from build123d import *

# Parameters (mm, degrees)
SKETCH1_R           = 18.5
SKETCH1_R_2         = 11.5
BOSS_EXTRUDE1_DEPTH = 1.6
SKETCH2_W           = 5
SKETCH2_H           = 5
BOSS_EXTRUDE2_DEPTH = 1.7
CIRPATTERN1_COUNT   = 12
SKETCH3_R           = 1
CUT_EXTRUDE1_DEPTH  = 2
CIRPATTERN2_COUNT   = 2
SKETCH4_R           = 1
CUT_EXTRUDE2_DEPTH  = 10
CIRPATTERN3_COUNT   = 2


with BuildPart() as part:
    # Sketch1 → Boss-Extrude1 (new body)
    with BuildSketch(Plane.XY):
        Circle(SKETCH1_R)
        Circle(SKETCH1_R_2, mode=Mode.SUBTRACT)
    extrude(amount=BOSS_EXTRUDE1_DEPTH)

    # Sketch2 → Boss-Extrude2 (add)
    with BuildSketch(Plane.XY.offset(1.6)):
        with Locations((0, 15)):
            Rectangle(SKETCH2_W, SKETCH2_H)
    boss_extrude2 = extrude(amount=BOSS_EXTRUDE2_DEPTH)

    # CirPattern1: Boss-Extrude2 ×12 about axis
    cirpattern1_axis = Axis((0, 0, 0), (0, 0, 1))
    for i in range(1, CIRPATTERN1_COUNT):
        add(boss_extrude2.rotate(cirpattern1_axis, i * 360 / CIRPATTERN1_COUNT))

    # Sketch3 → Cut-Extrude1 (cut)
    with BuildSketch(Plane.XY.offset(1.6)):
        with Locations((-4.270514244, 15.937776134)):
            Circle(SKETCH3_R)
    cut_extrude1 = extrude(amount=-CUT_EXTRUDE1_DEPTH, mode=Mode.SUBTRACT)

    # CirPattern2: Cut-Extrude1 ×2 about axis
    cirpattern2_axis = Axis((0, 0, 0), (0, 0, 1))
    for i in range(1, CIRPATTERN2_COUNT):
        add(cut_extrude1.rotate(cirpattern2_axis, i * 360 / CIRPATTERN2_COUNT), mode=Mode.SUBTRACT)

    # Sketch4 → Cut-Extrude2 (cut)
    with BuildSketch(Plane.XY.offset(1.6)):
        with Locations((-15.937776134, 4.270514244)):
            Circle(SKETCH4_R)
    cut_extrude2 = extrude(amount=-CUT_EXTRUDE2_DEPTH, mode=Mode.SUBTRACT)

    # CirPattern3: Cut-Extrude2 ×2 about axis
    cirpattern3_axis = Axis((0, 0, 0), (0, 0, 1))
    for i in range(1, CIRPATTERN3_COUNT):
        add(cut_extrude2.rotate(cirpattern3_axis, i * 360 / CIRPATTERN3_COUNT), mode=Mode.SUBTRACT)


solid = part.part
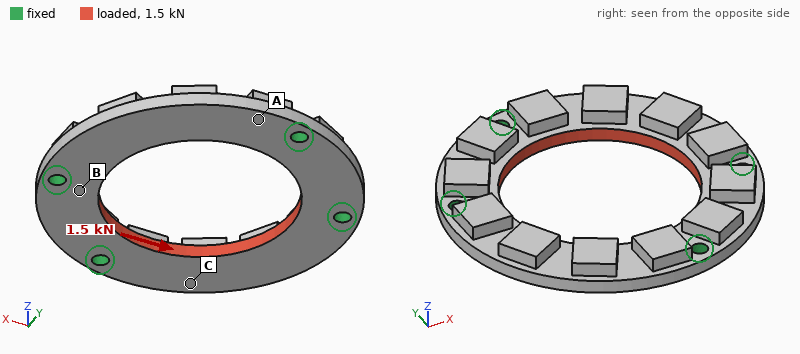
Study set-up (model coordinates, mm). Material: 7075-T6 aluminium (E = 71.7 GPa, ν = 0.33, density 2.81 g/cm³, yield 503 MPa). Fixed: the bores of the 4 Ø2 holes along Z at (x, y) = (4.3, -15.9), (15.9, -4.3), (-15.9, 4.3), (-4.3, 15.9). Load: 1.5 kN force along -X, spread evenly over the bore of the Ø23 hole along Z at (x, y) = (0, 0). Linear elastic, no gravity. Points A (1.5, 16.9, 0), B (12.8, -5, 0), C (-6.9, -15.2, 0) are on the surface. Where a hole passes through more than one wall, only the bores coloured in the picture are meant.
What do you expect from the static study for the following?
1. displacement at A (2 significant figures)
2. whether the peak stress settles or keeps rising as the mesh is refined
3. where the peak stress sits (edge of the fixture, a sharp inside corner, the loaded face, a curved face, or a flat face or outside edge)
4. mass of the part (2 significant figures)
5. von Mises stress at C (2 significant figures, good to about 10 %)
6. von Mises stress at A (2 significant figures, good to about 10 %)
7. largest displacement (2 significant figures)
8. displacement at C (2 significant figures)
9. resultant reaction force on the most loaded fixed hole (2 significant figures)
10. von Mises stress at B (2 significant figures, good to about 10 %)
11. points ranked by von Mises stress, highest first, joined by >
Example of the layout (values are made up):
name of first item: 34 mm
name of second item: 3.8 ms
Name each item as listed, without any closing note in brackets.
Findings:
displacement at A: 2.1 µm
whether the peak stress settles or keeps rising as the mesh is refined: keeps rising
where the peak stress sits: edge of the fixture
mass of the part: 4.3 g
von Mises stress at C: 18 MPa
von Mises stress at A: 26 MPa
largest displacement: 8.5 µm
displacement at C: 4.5 µm
resultant reaction force on the most loaded fixed hole: 430 N
von Mises stress at B: 39 MPa
points ranked by von Mises stress, highest first, joined by >: B > A > C
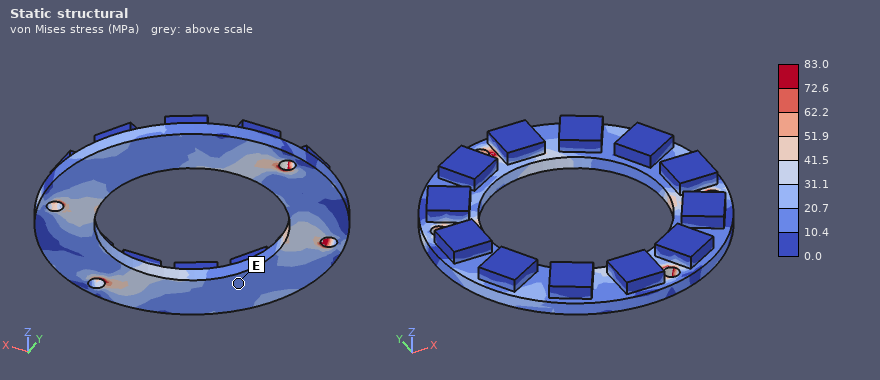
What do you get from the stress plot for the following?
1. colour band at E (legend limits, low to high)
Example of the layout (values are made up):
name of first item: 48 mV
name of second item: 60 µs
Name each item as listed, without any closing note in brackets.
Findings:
colour band at E: 10.4 to 20.7 MPa
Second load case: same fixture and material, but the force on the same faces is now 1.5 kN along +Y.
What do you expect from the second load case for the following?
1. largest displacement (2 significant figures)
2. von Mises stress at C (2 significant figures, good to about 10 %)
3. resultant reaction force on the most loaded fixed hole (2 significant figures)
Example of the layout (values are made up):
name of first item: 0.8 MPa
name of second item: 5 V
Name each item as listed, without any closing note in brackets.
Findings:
largest displacement: 8.5 µm
von Mises stress at C: 20 MPa
resultant reaction force on the most loaded fixed hole: 430 N
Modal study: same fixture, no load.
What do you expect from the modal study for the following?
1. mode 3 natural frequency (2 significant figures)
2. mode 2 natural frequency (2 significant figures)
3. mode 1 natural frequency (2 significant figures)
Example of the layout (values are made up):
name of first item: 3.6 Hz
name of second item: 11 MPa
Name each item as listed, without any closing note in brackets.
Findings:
mode 3 natural frequency: 20 kHz
mode 2 natural frequency: 7400 Hz
mode 1 natural frequency: 7300 Hz
